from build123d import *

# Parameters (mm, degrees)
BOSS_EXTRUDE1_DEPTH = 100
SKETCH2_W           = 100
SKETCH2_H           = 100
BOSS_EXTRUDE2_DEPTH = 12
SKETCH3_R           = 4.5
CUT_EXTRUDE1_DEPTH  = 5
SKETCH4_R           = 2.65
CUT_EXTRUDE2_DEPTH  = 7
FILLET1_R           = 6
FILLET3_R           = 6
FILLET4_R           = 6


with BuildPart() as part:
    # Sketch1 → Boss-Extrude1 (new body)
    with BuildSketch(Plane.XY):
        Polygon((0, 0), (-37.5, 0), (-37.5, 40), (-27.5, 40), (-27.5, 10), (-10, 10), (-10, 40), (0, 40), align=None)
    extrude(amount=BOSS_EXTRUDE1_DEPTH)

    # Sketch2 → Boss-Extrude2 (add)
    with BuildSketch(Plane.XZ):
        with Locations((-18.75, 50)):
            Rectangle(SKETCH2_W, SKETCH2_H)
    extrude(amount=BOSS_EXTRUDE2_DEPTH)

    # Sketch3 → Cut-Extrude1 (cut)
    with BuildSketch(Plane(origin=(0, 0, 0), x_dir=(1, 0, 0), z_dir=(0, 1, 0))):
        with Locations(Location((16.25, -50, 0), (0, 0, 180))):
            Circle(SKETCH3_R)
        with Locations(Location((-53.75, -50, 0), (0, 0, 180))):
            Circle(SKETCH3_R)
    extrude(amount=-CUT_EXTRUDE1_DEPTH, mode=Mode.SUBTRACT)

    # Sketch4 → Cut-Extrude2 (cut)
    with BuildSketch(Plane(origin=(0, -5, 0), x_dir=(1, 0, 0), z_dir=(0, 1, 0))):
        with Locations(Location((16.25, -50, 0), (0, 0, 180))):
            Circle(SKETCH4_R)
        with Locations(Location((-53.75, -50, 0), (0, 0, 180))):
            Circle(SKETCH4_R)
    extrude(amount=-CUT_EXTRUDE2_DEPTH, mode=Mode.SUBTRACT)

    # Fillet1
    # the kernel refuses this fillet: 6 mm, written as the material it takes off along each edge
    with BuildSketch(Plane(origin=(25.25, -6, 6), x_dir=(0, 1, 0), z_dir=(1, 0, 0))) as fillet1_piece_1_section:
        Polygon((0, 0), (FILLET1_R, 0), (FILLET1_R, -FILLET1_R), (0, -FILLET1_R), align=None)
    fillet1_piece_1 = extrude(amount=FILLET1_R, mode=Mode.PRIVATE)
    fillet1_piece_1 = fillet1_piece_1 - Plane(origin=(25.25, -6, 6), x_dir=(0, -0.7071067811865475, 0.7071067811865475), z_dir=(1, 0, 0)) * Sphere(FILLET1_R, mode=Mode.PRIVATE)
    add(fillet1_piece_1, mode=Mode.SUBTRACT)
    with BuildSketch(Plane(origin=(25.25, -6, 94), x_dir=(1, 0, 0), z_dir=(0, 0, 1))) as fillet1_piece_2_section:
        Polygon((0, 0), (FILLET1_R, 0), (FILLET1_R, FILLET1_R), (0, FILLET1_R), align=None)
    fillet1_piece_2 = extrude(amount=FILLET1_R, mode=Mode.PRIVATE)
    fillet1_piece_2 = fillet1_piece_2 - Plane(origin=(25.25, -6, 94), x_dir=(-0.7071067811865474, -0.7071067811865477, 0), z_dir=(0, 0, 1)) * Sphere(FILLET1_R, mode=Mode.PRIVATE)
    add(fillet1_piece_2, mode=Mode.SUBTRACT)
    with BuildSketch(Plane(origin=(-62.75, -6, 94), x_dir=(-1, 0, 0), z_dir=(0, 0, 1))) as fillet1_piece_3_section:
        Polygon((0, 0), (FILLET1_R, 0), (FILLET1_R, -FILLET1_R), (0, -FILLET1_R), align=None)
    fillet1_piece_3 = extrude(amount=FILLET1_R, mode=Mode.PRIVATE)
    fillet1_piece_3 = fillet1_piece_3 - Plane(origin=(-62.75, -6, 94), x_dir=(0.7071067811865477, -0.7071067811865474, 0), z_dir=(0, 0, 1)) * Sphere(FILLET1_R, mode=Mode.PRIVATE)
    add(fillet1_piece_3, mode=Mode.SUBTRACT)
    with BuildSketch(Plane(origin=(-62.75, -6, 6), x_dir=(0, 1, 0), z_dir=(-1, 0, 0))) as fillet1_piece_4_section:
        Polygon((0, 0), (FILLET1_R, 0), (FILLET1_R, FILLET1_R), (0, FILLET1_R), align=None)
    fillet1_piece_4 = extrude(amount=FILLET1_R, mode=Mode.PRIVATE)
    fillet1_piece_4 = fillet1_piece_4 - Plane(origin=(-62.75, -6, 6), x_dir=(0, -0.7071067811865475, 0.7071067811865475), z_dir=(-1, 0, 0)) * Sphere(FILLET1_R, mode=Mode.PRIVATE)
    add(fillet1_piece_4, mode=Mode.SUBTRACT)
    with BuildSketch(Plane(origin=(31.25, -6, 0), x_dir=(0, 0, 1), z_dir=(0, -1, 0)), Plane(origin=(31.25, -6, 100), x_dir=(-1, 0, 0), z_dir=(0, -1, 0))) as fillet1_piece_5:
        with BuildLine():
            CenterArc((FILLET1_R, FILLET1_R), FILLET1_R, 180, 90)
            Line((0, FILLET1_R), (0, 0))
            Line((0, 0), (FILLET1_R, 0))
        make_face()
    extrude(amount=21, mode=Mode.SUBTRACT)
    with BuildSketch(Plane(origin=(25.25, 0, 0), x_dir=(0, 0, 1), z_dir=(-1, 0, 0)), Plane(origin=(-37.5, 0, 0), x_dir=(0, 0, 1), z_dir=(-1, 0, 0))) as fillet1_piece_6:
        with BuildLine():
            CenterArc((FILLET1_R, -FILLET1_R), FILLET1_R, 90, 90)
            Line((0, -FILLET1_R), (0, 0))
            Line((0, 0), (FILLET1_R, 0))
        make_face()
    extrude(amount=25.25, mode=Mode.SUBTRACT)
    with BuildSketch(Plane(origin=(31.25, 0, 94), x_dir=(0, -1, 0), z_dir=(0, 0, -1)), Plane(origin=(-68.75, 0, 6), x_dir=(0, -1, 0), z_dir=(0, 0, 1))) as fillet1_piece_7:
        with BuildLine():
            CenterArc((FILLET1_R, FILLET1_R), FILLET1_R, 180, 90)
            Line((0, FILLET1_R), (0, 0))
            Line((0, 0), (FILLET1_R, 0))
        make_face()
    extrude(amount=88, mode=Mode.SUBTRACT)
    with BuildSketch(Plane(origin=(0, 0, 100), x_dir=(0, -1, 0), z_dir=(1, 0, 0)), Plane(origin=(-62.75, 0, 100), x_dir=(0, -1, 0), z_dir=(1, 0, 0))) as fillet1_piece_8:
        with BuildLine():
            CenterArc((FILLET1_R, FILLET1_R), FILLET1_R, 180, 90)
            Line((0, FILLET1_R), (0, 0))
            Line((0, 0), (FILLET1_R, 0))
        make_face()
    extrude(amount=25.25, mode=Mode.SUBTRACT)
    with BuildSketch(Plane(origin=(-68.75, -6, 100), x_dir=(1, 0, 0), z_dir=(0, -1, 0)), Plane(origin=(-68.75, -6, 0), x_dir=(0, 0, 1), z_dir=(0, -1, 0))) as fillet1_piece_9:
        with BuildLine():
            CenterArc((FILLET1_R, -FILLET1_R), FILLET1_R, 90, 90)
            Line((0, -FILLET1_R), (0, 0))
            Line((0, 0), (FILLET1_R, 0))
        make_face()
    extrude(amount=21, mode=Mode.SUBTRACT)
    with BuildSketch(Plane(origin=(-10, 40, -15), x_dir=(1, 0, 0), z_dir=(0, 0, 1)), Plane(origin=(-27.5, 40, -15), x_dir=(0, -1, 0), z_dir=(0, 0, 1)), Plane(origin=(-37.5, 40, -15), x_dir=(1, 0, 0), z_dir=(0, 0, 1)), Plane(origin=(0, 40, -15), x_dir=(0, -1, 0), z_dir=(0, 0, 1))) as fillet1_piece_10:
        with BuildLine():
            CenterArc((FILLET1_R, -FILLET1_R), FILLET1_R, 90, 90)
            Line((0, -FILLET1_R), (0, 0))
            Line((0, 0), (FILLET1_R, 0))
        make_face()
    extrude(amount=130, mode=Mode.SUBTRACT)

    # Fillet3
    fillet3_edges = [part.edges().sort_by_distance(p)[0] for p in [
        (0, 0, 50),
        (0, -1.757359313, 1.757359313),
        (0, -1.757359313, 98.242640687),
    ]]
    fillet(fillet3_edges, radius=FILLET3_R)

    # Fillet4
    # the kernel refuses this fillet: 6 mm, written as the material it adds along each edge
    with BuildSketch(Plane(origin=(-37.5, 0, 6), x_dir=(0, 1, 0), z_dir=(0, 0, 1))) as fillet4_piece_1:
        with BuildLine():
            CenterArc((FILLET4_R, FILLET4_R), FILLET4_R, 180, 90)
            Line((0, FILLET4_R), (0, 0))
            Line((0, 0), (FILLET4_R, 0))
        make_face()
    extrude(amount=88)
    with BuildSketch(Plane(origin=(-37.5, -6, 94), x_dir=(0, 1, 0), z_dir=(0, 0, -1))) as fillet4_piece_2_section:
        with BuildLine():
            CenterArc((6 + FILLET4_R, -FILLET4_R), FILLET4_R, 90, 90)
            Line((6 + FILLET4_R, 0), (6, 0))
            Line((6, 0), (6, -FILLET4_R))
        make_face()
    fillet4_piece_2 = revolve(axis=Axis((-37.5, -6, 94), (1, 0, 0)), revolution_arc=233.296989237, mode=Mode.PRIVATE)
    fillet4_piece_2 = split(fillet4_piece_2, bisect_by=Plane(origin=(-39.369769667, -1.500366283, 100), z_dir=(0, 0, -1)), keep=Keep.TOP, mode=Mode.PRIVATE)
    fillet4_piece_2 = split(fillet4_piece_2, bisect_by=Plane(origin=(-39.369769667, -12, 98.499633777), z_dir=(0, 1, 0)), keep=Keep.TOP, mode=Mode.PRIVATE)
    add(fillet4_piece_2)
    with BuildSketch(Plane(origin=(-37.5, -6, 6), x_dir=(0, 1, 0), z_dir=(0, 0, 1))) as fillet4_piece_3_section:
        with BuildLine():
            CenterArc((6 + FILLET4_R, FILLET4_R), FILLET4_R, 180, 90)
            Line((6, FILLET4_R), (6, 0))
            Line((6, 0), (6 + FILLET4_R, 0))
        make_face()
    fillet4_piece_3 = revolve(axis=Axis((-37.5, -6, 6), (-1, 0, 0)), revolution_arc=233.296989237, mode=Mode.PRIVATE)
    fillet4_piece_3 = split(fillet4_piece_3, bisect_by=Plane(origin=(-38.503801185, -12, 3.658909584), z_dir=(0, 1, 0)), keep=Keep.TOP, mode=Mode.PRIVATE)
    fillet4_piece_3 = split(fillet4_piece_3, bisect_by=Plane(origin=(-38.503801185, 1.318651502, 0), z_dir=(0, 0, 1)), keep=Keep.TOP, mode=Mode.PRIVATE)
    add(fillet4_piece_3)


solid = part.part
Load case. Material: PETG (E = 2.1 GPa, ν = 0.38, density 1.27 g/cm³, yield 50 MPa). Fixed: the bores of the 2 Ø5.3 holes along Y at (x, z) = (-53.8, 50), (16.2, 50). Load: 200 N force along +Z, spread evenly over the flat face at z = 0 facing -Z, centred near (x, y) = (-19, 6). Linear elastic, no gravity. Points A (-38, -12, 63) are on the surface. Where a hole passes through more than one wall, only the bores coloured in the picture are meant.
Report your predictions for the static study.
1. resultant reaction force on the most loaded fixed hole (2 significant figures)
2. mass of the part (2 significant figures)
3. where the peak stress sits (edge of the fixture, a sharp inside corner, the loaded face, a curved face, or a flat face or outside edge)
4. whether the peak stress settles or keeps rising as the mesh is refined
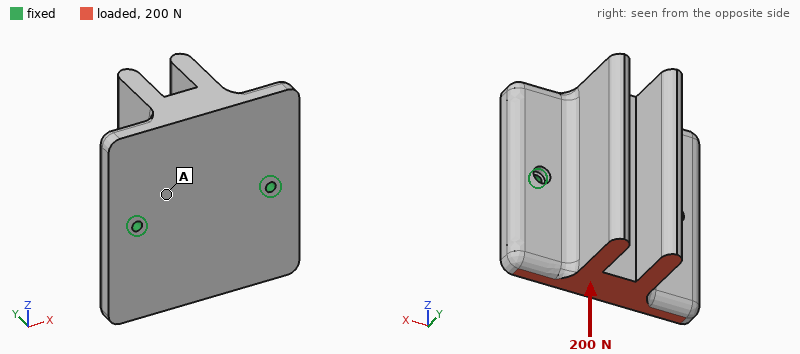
100 N
270 g
edge of the fixture
keeps rising
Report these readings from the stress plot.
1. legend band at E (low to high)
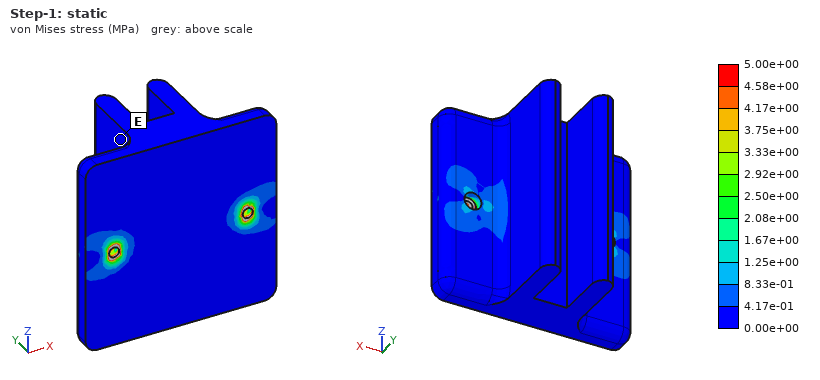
0.00e+00 to 4.17e-01 MPa
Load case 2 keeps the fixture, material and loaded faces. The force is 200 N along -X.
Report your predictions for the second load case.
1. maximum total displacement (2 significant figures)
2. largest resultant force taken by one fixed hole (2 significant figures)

75 µm
180 N
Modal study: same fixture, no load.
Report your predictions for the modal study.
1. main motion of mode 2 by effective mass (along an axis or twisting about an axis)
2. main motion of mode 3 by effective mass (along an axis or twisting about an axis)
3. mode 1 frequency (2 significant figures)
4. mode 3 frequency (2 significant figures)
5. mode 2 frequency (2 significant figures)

along Y
along X
260 Hz
1200 Hz
1100 Hz
